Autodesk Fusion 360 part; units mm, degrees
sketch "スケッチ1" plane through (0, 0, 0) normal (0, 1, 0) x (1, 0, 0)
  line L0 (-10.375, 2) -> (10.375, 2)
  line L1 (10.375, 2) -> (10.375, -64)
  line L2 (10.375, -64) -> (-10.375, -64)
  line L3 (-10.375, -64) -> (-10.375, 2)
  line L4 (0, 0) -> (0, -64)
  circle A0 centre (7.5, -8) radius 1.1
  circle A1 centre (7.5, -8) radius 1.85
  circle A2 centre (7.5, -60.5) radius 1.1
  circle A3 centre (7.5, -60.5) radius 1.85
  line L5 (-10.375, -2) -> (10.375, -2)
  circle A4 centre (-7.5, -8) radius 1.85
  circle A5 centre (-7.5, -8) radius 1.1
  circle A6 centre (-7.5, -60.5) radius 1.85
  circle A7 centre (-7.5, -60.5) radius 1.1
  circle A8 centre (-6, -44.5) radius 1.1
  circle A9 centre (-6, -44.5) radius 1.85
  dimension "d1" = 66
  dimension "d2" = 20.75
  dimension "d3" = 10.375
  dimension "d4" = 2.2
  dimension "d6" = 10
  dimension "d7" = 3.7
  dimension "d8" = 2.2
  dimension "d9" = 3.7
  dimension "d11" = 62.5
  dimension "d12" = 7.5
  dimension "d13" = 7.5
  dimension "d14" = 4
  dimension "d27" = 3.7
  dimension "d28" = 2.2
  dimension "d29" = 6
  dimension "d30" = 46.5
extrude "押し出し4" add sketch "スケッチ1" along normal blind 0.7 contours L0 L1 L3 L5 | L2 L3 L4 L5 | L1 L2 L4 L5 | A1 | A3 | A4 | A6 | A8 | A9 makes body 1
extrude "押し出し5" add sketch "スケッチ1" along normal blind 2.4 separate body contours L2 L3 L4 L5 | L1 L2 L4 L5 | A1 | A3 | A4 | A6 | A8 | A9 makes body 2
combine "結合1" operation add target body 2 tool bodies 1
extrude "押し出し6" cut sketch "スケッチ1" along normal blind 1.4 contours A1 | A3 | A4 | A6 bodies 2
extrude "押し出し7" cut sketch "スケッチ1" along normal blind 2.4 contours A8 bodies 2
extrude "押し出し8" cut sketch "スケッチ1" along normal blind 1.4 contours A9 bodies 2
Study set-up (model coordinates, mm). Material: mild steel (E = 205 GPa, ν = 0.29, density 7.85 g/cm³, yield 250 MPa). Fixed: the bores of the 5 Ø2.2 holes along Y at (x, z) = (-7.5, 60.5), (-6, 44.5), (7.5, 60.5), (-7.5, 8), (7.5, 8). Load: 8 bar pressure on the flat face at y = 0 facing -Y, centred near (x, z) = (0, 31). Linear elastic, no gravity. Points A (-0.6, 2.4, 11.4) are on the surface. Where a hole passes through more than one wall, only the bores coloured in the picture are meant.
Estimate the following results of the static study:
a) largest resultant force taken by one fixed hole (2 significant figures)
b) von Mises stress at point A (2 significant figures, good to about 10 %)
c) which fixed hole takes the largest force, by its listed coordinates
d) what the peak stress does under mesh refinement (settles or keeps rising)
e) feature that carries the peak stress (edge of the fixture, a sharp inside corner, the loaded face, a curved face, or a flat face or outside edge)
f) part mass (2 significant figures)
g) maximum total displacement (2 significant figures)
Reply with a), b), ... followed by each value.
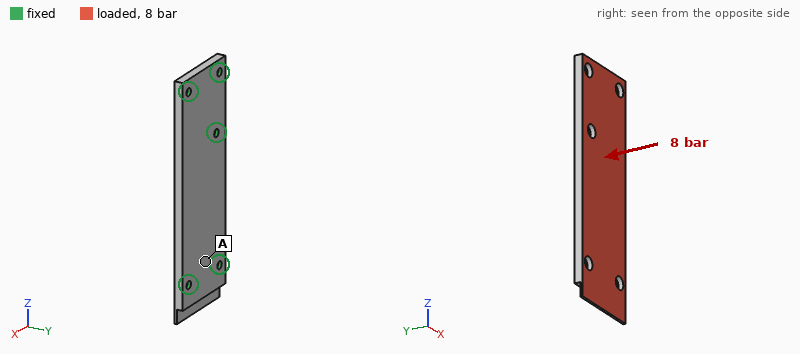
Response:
a) 520 N
b) 44 MPa
c) (-6, 44.5)
d) keeps rising
e) edge of the fixture
f) 24 g
g) 48 µm
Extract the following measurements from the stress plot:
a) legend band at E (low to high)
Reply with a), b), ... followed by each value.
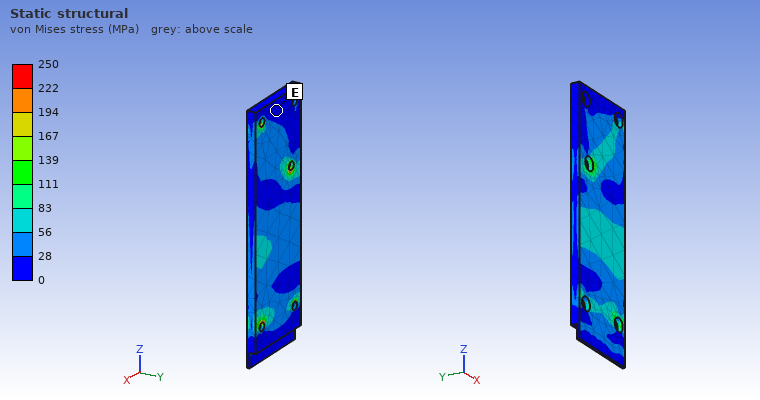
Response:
a) 0 to 28 MPa
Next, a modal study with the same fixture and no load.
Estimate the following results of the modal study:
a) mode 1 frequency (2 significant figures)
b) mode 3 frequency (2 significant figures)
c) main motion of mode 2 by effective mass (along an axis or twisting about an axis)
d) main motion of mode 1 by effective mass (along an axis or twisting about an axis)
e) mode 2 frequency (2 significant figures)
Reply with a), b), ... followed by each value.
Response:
a) 6000 Hz
b) 15 kHz
c) twisting about Z
d) along Y
e) 9700 Hz
